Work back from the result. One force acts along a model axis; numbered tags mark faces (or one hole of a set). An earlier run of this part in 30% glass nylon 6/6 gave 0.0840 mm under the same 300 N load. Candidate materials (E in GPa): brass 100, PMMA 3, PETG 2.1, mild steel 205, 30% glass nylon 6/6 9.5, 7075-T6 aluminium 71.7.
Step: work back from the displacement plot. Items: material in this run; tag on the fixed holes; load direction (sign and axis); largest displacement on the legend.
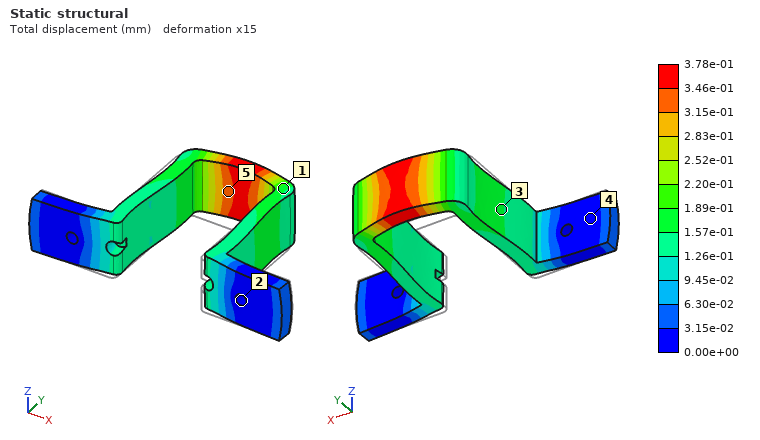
PETG
2
+Y
3.78e-01 mm
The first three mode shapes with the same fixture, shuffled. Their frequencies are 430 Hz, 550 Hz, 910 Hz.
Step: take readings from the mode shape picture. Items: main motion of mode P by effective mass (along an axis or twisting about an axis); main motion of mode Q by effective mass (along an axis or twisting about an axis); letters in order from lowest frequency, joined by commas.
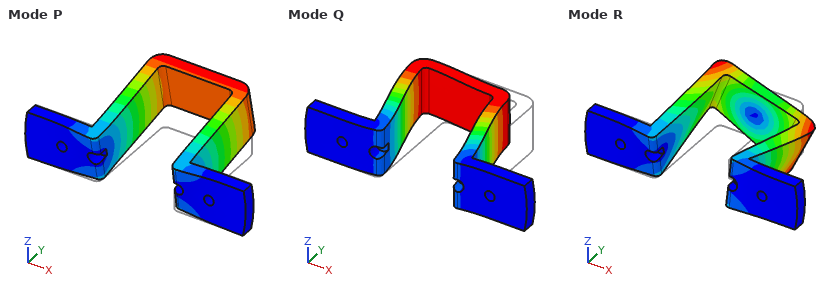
along Z
along X
P, Q, R
